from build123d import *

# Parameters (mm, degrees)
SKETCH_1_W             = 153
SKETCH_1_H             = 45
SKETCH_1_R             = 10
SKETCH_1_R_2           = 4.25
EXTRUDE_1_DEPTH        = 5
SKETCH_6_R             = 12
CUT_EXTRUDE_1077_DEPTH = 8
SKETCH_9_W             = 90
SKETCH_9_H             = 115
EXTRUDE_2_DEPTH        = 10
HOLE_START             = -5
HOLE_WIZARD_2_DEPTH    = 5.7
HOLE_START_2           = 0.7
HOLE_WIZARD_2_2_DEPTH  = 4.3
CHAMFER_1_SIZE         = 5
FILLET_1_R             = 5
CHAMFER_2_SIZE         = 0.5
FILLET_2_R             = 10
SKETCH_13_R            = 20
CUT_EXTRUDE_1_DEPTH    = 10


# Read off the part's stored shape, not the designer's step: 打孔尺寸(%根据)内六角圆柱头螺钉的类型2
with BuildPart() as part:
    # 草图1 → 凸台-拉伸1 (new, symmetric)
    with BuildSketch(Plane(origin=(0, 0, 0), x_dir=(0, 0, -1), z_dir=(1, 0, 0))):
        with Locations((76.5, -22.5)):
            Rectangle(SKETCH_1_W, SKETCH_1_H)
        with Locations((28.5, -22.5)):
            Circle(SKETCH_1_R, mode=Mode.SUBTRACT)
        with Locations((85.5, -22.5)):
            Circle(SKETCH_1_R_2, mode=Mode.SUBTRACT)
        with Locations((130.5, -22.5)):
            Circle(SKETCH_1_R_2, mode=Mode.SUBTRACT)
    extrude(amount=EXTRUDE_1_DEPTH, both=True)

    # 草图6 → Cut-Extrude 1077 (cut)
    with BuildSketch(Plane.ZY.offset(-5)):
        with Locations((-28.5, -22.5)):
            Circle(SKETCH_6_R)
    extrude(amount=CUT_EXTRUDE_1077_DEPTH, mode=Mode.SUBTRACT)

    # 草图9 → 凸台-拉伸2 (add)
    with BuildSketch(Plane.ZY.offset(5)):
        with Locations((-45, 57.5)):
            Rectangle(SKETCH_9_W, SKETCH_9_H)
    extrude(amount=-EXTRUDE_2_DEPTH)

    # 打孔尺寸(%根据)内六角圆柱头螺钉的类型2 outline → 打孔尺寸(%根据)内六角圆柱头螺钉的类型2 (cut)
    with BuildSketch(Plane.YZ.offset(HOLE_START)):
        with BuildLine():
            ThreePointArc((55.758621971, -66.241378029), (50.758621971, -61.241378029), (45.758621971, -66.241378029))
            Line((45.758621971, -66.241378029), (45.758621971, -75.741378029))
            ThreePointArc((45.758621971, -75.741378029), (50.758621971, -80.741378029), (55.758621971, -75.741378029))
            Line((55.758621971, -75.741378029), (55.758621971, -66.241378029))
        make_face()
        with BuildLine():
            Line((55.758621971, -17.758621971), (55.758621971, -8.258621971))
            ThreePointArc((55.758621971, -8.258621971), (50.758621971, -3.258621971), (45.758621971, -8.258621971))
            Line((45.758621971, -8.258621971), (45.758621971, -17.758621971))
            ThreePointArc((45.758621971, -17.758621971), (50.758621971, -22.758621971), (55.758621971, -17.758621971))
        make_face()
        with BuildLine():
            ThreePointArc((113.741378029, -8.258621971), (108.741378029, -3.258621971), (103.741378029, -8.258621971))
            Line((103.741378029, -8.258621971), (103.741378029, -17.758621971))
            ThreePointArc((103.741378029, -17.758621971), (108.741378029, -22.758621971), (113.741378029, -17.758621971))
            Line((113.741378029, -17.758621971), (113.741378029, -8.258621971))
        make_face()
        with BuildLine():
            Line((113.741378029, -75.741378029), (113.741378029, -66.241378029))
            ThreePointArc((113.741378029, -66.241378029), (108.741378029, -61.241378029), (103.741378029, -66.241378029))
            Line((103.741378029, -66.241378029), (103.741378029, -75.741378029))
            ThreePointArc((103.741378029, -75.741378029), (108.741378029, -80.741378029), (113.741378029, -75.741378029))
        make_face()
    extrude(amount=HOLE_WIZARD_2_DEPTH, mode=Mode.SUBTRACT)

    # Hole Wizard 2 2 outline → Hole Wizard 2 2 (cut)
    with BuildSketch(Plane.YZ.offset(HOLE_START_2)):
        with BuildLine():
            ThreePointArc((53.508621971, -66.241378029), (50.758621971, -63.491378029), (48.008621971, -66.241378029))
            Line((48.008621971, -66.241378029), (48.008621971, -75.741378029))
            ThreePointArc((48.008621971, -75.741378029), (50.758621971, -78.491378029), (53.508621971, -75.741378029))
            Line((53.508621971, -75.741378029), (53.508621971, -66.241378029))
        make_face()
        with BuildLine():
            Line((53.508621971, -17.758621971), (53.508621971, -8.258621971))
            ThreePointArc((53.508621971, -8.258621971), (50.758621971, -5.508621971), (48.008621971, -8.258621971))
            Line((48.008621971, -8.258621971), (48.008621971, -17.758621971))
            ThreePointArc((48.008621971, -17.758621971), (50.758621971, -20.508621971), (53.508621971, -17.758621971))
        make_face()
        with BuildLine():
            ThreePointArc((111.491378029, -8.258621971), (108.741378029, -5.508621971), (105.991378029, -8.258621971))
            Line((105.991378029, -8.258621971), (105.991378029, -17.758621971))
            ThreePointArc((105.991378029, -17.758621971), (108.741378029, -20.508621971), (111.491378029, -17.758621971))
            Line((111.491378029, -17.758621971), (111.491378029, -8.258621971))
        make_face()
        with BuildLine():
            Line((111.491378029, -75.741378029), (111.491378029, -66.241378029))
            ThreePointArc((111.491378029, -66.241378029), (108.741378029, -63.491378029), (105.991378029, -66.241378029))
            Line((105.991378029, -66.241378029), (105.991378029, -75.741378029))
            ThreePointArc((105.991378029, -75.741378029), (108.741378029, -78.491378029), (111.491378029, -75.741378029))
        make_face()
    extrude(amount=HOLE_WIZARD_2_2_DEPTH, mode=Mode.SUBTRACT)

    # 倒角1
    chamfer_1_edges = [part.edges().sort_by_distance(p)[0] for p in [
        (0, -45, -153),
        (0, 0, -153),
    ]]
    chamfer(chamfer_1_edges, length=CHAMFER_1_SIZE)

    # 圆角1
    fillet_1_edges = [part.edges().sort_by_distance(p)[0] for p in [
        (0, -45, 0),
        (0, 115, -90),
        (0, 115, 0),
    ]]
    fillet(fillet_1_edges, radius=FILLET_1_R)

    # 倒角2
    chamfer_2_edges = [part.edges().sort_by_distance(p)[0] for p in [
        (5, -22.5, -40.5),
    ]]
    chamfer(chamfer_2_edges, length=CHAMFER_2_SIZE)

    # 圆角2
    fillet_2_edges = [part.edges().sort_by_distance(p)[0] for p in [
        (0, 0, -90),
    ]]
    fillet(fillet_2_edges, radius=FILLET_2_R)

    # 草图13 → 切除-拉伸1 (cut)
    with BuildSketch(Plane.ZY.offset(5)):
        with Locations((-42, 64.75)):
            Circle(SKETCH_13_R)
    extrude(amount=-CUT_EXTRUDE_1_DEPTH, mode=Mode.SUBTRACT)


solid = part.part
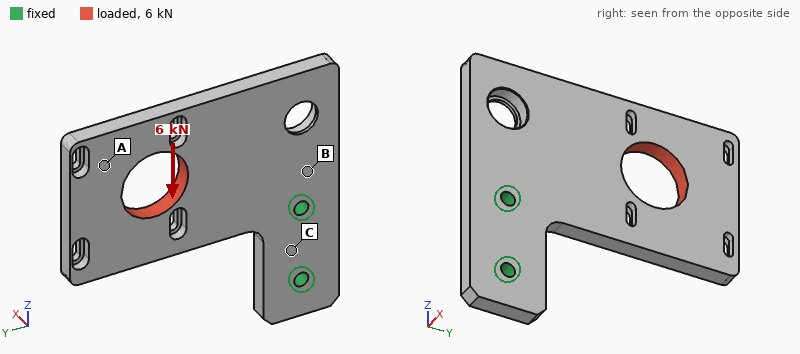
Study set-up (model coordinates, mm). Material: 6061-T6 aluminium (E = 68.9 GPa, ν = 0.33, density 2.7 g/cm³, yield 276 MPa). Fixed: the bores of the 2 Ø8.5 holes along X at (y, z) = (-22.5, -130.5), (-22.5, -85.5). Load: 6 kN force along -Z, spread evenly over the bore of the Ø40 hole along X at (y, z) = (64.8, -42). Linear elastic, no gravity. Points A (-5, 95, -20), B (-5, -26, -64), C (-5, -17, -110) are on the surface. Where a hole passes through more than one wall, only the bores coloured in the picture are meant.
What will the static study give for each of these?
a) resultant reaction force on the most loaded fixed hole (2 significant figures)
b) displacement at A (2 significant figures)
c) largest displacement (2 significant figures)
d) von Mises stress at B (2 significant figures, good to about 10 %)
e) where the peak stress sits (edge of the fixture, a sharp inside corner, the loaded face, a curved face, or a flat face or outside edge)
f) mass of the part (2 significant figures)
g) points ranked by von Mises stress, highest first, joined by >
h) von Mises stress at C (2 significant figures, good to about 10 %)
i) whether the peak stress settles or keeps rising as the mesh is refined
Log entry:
9.7 kN
0.53 mm
0.63 mm
41 MPa
edge of the fixture
400 g
C > B > A
55 MPa
keeps rising
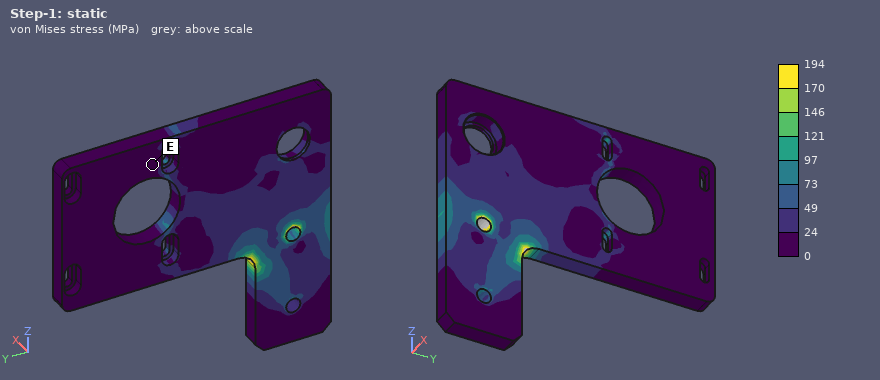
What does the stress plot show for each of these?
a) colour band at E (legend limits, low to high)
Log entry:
0 to 24 MPa
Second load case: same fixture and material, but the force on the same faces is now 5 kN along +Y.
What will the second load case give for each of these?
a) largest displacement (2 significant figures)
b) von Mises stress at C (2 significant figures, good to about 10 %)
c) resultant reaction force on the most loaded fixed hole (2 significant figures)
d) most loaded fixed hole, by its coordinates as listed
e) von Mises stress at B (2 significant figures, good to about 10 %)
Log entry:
0.25 mm
20 MPa
8.6 kN
(-22.5, -85.5)
21 MPa
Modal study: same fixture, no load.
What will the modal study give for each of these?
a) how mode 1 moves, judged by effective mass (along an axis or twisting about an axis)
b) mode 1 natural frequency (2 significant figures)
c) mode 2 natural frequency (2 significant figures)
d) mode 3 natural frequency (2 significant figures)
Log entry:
along X
340 Hz
820 Hz
1200 Hz
